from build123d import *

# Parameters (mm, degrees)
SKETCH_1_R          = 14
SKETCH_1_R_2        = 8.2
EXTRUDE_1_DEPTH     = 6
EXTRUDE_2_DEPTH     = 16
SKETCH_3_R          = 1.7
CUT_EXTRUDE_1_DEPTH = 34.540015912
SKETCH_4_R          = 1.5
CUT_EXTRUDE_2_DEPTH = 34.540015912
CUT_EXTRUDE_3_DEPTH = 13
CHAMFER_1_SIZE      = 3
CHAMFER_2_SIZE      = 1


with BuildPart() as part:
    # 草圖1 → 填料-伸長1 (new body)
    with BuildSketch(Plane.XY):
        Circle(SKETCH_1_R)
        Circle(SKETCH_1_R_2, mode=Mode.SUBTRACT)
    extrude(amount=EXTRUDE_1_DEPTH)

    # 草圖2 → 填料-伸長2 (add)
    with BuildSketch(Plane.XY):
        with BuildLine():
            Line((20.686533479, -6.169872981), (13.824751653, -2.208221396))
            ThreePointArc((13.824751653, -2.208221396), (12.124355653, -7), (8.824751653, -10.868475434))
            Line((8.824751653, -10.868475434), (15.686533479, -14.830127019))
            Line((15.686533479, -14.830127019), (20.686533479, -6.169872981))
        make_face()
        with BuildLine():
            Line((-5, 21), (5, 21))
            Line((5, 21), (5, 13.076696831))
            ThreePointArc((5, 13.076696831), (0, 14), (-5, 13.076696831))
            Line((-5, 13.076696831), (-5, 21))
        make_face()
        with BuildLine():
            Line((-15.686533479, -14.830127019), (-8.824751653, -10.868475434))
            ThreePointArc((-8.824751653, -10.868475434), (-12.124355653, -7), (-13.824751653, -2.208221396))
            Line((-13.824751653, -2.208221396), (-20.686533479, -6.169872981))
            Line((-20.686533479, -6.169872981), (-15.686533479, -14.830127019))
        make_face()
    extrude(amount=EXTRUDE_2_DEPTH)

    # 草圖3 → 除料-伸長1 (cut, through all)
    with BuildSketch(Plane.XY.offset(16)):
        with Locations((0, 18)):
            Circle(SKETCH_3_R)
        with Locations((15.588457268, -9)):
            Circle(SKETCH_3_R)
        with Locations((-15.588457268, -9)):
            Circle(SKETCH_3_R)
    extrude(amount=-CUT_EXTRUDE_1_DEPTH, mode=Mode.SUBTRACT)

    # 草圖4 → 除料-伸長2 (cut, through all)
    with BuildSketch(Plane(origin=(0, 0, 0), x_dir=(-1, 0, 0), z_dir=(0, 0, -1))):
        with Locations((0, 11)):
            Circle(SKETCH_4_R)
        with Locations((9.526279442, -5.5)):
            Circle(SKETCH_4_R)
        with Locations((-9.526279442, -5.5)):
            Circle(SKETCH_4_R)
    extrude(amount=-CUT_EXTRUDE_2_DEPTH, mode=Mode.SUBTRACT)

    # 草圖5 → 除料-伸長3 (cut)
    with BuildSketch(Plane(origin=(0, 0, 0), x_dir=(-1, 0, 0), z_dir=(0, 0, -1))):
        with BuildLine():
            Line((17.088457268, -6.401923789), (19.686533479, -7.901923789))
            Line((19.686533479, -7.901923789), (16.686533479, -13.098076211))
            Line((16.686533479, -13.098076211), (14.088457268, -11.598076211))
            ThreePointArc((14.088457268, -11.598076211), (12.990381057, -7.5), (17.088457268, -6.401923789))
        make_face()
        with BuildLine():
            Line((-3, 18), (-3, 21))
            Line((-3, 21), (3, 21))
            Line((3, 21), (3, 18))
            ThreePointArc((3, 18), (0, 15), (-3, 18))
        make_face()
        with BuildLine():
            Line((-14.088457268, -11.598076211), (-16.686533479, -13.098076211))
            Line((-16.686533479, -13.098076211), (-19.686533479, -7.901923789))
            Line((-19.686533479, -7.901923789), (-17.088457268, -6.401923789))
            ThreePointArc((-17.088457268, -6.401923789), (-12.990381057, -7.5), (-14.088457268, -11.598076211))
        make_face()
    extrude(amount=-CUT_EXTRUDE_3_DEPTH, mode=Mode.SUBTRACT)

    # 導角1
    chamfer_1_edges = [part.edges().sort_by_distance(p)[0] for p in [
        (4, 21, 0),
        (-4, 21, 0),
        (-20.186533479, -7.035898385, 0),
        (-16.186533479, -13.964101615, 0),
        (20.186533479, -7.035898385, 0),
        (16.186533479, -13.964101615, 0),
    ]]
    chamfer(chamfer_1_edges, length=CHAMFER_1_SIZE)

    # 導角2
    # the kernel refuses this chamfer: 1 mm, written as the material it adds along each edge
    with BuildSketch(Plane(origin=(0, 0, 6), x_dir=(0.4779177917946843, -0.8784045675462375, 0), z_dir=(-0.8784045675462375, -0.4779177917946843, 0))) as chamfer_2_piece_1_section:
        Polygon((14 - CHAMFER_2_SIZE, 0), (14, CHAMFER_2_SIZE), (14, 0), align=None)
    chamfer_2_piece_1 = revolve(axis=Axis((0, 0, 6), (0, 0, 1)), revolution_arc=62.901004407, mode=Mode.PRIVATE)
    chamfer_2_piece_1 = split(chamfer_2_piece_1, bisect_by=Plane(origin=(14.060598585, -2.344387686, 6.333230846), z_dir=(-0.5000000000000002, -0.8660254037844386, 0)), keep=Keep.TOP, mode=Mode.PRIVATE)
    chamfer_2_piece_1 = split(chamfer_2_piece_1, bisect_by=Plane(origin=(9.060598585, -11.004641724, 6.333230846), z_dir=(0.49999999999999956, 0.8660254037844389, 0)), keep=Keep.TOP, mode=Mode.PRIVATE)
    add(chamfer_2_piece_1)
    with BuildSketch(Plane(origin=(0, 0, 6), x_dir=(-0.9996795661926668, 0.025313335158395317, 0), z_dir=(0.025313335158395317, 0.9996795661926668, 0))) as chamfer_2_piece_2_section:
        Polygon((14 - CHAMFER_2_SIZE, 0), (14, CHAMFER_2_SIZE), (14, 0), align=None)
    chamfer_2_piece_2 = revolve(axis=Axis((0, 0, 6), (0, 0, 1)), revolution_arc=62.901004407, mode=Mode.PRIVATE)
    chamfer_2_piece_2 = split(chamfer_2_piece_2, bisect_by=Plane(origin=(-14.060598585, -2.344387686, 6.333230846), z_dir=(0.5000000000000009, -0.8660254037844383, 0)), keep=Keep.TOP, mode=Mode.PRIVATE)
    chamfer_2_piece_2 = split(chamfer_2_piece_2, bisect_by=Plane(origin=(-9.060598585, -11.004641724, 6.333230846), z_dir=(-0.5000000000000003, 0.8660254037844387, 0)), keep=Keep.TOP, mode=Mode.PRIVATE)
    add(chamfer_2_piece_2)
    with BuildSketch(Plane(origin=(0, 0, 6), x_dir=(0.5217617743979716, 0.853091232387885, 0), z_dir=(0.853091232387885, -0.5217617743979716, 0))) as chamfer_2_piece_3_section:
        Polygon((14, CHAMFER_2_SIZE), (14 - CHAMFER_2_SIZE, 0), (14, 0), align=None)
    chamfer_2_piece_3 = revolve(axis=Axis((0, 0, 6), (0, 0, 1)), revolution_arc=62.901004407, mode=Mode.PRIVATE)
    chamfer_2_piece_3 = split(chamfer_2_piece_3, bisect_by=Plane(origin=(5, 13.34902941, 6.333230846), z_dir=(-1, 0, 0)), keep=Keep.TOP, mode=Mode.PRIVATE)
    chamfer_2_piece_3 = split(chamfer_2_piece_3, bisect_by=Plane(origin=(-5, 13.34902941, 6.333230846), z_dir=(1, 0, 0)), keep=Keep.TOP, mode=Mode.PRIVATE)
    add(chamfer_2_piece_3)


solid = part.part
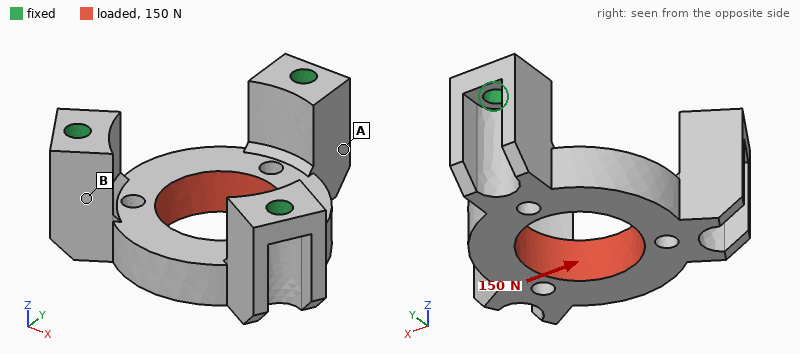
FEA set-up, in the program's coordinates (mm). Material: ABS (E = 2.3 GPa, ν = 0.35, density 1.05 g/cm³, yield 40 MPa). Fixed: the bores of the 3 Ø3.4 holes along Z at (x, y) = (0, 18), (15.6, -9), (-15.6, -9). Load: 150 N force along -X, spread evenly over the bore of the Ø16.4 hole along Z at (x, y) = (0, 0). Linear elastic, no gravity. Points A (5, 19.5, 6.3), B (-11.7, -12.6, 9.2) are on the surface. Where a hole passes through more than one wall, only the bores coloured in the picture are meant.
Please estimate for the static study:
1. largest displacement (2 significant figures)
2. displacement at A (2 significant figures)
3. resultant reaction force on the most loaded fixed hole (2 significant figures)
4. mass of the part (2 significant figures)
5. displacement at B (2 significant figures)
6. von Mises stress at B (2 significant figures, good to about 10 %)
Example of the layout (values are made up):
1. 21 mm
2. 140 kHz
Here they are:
1. 0.11 mm
2. 0.063 mm
3. 63 N
4. 4.7 g
5. 0.040 mm
6. 3.1 MPa
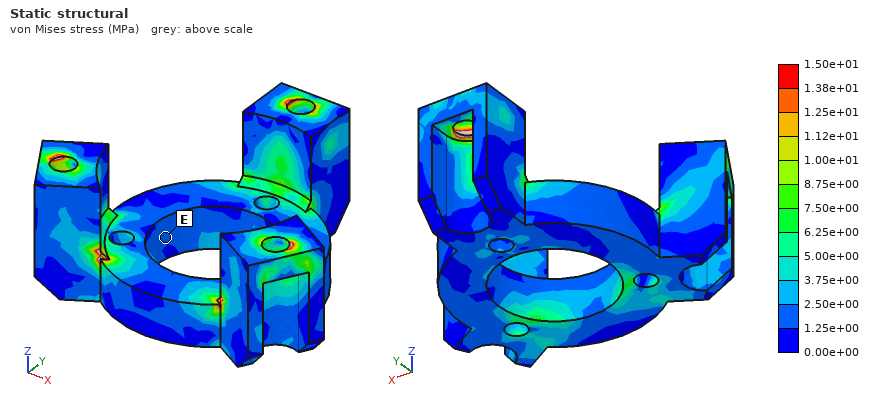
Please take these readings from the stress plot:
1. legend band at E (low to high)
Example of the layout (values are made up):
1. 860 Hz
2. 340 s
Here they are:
1. 1.25e+00 to 2.50e+00 MPa
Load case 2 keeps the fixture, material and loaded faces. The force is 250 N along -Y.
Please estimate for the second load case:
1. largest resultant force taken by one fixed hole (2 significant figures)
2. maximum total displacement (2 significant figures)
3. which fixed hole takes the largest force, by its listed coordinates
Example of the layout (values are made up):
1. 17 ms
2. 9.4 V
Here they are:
1. 110 N
2. 0.19 mm
3. (0, 18)
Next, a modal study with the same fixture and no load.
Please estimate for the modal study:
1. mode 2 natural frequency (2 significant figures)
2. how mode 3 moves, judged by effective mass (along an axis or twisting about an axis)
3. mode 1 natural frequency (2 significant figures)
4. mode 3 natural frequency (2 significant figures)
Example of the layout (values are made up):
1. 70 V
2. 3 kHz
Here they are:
1. 3600 Hz
2. twisting about Z
3. 3600 Hz
4. 4200 Hz
